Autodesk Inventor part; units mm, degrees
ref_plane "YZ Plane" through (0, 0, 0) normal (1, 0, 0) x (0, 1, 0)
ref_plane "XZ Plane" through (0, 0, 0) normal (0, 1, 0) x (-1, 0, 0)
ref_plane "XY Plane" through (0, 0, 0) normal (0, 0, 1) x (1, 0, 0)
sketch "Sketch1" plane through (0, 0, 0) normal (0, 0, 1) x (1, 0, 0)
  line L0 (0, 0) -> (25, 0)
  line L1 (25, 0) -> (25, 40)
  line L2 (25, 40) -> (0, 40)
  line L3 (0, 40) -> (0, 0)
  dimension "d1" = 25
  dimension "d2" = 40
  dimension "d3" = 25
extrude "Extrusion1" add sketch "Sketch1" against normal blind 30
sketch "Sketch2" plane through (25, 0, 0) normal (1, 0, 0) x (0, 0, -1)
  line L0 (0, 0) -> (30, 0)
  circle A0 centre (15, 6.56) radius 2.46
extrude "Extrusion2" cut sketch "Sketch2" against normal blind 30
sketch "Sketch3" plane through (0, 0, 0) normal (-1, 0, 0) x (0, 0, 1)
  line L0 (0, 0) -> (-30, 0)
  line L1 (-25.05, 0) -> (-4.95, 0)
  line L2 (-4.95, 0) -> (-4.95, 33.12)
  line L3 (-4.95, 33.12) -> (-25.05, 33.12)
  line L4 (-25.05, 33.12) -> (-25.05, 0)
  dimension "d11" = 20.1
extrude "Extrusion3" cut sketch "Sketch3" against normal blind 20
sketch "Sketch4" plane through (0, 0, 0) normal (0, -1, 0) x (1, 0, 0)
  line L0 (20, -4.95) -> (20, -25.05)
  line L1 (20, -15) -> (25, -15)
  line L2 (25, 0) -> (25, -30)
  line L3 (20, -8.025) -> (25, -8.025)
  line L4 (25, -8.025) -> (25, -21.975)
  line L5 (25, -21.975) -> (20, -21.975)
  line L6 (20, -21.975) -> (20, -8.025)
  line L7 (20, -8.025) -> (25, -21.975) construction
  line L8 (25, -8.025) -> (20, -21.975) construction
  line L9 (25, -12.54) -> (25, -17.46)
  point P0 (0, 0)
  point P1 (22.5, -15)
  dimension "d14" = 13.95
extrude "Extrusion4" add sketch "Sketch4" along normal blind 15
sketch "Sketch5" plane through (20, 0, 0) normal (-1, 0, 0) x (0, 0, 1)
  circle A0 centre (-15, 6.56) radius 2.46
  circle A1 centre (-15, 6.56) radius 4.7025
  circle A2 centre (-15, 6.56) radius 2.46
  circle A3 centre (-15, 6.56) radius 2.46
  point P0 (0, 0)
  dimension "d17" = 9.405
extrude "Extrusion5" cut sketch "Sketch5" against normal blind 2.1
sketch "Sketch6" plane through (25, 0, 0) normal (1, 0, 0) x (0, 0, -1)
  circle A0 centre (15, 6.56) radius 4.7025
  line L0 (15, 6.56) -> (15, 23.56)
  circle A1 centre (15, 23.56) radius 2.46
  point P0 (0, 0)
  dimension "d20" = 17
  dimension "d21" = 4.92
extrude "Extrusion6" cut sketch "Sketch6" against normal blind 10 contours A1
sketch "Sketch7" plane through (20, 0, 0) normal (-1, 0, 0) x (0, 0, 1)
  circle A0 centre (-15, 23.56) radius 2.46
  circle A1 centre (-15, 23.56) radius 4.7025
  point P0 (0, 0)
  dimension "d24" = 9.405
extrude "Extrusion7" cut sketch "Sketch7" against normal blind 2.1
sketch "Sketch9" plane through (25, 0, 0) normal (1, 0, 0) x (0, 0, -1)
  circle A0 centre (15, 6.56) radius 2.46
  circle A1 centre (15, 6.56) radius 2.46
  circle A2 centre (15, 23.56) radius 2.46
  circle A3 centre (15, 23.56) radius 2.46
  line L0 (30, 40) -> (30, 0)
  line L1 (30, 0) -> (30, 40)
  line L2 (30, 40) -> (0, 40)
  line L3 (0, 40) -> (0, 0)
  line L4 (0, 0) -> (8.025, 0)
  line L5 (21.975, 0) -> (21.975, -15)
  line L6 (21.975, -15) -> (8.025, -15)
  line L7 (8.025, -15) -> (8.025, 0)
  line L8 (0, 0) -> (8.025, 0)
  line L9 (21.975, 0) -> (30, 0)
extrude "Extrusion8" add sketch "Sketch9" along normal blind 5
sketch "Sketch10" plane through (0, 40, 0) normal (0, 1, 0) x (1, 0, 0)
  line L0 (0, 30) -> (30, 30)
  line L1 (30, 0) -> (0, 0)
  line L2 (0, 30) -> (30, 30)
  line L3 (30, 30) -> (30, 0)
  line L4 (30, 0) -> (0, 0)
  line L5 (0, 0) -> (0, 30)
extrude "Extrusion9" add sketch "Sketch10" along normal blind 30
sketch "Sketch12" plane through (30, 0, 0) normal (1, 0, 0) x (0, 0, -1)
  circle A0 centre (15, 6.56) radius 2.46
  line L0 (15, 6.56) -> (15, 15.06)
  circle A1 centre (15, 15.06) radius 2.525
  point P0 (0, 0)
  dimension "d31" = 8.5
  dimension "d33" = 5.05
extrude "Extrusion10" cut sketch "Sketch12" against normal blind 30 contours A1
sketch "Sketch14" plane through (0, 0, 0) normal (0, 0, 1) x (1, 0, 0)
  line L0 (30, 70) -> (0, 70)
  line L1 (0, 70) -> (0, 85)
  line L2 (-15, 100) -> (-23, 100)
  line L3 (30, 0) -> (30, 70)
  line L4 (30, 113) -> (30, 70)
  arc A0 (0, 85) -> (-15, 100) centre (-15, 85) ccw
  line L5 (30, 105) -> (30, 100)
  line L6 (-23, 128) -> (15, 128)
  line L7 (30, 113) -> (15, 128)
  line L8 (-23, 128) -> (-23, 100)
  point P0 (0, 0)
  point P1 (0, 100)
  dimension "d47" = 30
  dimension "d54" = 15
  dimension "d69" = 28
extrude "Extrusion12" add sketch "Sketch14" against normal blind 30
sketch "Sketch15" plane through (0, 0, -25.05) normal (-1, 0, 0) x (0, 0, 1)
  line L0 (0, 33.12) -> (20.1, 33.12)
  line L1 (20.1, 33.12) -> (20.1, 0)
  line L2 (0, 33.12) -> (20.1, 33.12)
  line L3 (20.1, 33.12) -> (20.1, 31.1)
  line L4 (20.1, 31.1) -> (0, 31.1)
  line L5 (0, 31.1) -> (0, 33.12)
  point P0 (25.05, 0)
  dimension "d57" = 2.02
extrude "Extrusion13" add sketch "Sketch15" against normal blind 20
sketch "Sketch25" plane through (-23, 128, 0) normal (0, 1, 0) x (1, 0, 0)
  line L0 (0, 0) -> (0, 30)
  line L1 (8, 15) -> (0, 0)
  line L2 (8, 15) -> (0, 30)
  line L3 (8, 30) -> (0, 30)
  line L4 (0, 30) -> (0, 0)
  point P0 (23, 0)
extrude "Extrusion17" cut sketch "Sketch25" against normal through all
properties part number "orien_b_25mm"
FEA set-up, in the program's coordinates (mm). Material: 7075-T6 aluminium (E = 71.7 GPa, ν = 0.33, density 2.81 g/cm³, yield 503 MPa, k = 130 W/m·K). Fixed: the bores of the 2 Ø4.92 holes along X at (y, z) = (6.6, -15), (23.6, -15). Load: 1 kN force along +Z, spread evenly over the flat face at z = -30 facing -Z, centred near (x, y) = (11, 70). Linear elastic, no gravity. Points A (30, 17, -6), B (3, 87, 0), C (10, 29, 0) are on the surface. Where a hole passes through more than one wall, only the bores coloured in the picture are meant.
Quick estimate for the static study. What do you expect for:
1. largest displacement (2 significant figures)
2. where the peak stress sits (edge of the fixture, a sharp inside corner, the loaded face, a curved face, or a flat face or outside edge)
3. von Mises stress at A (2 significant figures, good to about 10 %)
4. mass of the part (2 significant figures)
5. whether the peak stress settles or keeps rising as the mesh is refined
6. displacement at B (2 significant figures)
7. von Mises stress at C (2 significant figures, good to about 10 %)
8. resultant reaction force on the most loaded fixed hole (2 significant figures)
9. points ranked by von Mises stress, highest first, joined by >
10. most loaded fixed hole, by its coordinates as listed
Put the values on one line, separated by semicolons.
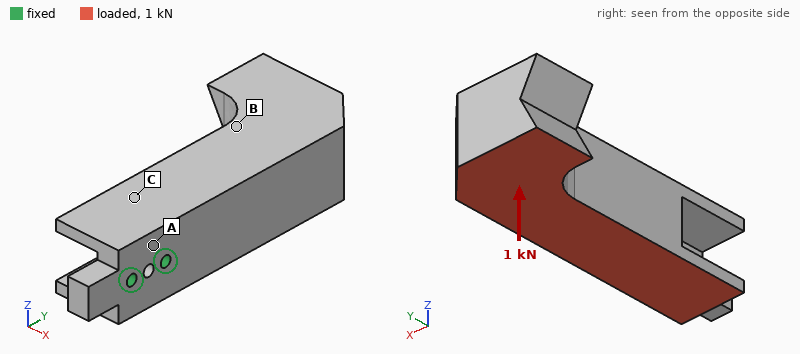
0.12 mm; edge of the fixture; 19 MPa; 330 g; keeps rising; 0.066 mm; 12 MPa; 3.0 kN; A > C > B; (23.6, -15)
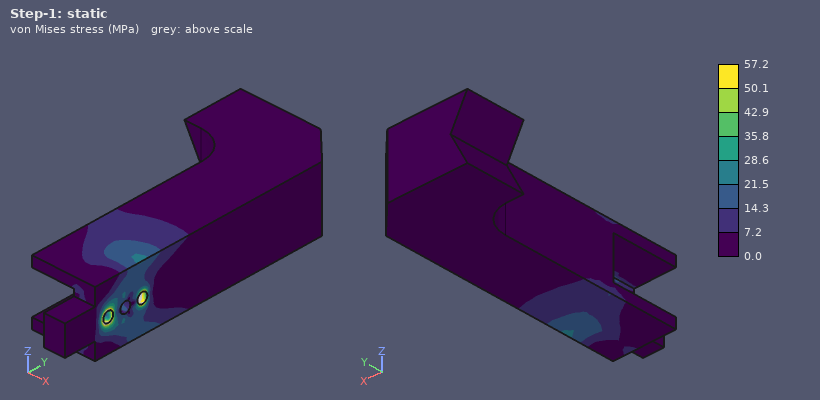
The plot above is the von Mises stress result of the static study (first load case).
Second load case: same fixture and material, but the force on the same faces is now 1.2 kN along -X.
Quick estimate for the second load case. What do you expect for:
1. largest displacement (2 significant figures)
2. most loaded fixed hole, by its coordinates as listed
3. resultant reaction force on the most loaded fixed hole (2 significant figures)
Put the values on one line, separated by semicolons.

0.19 mm; (23.6, -15); 3.3 kN
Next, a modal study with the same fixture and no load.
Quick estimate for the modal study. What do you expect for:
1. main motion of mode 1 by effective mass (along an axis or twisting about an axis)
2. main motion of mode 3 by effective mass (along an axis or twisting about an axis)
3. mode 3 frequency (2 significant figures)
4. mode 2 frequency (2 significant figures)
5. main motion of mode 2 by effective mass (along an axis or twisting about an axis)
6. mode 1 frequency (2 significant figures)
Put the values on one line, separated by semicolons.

along X; twisting about Y; 2700 Hz; 990 Hz; along Z; 840 Hz
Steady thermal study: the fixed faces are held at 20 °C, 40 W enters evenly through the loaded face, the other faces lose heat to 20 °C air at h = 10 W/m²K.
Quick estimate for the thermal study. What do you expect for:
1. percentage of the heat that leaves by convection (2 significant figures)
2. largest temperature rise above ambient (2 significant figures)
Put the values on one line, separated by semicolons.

6.1 %; 25 K
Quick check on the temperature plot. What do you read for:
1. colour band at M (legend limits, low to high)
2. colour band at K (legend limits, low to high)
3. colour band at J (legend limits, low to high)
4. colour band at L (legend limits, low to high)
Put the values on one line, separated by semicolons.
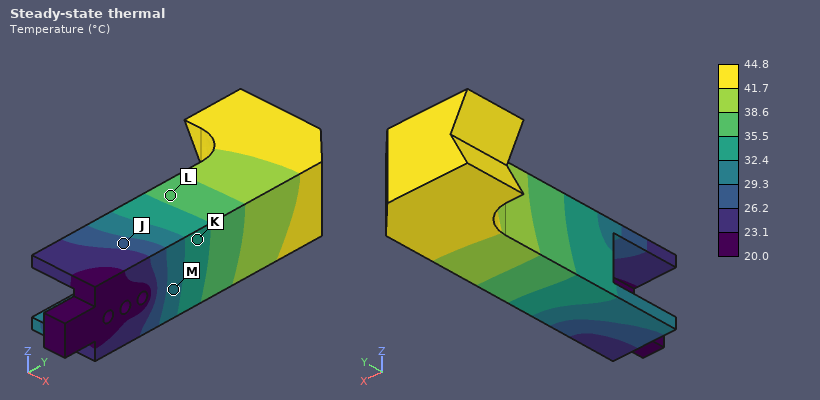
29.3 to 32.4 °C; 32.4 to 35.5 °C; 26.2 to 29.3 °C; 35.5 to 38.6 °C
